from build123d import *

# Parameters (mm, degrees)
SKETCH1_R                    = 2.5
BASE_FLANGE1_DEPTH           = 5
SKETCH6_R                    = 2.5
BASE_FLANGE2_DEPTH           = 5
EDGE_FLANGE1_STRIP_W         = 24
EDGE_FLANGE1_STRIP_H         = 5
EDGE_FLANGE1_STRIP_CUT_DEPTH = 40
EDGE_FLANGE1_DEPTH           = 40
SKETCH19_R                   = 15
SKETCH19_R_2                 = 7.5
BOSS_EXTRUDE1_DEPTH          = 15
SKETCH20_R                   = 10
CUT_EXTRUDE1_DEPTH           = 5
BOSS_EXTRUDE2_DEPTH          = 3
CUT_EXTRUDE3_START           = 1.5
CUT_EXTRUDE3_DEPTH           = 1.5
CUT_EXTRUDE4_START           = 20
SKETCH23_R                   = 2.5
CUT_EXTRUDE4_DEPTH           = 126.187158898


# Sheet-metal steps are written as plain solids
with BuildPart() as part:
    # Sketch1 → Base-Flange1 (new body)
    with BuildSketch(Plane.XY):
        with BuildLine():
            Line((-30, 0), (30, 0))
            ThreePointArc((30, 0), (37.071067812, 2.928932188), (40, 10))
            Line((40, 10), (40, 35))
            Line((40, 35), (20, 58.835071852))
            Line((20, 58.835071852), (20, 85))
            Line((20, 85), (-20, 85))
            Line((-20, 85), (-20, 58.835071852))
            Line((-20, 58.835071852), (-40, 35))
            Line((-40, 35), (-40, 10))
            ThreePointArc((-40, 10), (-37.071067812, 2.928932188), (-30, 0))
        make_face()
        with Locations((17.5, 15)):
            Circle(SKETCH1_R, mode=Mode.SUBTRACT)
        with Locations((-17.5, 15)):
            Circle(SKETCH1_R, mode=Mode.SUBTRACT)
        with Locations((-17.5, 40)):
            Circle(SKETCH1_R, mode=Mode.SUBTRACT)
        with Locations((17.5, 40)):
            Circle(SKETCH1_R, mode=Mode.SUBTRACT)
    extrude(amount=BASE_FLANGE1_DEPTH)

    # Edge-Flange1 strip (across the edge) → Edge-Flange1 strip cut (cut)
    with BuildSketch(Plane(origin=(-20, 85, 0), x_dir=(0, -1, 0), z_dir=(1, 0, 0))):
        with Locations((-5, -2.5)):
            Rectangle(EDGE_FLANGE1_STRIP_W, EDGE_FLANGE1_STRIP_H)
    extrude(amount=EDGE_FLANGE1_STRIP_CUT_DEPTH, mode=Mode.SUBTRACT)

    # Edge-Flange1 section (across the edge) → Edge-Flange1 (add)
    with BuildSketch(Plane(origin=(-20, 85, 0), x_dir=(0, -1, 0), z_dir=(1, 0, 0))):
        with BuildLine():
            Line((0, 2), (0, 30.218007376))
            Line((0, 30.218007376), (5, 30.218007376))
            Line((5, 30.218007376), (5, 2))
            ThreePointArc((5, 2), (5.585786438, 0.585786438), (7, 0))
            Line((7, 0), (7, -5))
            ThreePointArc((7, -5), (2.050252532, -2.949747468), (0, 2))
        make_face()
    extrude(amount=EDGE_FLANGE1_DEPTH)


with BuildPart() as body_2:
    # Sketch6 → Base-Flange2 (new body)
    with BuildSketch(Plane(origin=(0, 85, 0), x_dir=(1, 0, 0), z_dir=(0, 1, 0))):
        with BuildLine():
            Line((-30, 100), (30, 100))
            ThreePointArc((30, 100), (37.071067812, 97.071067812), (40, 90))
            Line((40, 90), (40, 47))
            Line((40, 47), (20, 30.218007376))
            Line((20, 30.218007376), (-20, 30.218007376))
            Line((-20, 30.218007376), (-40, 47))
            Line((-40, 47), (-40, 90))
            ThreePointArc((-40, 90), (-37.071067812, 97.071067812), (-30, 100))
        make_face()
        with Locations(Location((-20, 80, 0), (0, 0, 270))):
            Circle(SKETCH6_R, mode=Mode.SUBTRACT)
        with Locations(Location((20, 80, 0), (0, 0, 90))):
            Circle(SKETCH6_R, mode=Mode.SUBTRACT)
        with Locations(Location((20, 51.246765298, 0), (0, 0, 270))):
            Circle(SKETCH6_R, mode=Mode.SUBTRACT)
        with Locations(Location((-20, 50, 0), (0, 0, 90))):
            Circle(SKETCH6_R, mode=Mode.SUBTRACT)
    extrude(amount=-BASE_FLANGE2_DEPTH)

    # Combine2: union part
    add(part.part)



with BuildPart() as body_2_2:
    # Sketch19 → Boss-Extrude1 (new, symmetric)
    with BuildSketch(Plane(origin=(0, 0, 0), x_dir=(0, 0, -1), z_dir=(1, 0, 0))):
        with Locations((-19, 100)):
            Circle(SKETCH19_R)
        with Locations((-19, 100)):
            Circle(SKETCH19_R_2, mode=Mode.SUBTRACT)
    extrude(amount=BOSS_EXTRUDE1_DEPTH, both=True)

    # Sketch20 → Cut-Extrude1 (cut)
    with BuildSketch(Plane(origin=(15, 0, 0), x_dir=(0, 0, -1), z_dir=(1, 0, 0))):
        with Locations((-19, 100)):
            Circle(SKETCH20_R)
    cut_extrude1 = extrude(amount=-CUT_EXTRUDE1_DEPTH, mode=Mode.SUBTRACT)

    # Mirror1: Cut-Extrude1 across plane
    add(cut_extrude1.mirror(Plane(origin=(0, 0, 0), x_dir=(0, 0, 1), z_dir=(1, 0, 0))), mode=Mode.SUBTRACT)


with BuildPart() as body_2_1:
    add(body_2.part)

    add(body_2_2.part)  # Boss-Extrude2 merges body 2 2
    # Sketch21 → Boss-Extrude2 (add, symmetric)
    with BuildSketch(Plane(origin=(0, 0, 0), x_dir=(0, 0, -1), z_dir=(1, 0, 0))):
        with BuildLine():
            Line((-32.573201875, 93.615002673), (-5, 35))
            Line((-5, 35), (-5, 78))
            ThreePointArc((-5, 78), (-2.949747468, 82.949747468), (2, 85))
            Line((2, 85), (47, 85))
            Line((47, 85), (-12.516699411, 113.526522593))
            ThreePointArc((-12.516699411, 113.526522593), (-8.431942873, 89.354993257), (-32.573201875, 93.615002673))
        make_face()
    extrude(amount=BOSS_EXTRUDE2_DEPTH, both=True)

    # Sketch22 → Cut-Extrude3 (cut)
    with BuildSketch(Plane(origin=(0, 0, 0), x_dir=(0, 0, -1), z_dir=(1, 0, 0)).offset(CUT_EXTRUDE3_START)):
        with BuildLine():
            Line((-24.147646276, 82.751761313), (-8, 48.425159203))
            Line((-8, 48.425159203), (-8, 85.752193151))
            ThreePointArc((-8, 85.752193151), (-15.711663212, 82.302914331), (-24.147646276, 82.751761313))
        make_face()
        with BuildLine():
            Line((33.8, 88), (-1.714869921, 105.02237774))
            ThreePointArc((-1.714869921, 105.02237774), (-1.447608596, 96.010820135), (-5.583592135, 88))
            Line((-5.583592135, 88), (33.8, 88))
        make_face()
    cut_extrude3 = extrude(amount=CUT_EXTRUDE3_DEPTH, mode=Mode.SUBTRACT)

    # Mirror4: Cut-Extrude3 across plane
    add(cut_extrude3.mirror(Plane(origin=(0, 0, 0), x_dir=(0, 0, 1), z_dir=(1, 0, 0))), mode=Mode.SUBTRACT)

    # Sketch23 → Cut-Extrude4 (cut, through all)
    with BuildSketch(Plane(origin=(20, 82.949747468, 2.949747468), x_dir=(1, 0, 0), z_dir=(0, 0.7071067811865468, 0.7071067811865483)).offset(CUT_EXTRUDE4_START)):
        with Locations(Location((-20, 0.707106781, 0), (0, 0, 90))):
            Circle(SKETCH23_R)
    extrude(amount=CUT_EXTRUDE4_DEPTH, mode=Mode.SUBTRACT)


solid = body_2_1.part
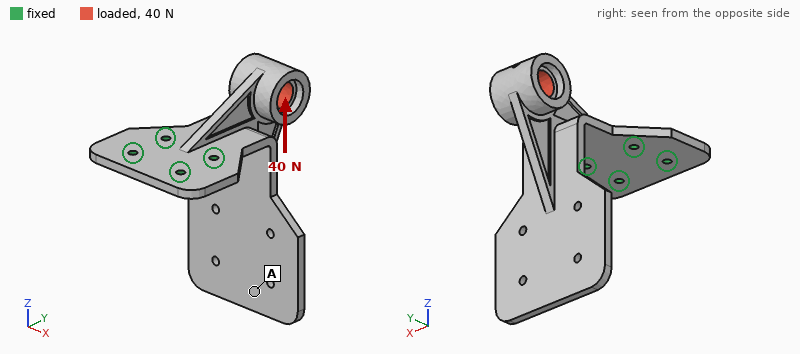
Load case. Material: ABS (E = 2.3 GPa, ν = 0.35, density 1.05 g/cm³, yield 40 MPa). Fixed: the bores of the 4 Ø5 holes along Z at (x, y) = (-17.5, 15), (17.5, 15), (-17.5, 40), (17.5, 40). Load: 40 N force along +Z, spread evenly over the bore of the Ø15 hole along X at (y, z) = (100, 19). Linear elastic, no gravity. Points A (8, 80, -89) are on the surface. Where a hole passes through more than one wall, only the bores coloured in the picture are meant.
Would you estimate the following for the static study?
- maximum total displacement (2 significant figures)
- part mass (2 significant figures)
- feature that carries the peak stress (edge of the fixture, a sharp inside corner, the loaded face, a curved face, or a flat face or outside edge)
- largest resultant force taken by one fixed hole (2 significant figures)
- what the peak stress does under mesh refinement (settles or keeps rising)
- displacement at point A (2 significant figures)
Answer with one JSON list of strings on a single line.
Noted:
["2.3 mm", "81 g", "edge of the fixture", "45 N", "keeps rising", "2.0 mm"]
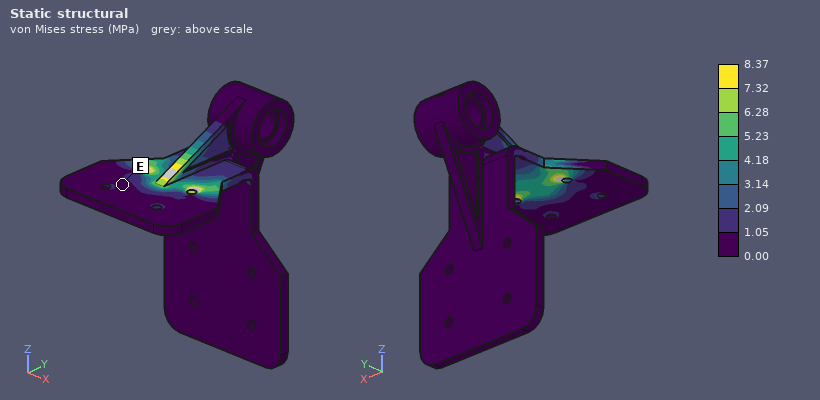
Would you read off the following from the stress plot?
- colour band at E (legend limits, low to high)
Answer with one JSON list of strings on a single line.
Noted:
["0.00 to 1.05 MPa"]
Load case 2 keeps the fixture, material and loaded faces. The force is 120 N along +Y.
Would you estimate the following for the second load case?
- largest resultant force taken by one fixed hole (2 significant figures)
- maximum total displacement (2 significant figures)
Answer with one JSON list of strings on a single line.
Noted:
["39 N", "2.1 mm"]
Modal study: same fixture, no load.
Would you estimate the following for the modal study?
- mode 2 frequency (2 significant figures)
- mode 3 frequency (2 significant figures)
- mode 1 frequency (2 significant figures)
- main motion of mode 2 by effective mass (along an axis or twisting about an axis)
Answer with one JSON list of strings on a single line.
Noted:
["100 Hz", "250 Hz", "93 Hz", "along X"]
